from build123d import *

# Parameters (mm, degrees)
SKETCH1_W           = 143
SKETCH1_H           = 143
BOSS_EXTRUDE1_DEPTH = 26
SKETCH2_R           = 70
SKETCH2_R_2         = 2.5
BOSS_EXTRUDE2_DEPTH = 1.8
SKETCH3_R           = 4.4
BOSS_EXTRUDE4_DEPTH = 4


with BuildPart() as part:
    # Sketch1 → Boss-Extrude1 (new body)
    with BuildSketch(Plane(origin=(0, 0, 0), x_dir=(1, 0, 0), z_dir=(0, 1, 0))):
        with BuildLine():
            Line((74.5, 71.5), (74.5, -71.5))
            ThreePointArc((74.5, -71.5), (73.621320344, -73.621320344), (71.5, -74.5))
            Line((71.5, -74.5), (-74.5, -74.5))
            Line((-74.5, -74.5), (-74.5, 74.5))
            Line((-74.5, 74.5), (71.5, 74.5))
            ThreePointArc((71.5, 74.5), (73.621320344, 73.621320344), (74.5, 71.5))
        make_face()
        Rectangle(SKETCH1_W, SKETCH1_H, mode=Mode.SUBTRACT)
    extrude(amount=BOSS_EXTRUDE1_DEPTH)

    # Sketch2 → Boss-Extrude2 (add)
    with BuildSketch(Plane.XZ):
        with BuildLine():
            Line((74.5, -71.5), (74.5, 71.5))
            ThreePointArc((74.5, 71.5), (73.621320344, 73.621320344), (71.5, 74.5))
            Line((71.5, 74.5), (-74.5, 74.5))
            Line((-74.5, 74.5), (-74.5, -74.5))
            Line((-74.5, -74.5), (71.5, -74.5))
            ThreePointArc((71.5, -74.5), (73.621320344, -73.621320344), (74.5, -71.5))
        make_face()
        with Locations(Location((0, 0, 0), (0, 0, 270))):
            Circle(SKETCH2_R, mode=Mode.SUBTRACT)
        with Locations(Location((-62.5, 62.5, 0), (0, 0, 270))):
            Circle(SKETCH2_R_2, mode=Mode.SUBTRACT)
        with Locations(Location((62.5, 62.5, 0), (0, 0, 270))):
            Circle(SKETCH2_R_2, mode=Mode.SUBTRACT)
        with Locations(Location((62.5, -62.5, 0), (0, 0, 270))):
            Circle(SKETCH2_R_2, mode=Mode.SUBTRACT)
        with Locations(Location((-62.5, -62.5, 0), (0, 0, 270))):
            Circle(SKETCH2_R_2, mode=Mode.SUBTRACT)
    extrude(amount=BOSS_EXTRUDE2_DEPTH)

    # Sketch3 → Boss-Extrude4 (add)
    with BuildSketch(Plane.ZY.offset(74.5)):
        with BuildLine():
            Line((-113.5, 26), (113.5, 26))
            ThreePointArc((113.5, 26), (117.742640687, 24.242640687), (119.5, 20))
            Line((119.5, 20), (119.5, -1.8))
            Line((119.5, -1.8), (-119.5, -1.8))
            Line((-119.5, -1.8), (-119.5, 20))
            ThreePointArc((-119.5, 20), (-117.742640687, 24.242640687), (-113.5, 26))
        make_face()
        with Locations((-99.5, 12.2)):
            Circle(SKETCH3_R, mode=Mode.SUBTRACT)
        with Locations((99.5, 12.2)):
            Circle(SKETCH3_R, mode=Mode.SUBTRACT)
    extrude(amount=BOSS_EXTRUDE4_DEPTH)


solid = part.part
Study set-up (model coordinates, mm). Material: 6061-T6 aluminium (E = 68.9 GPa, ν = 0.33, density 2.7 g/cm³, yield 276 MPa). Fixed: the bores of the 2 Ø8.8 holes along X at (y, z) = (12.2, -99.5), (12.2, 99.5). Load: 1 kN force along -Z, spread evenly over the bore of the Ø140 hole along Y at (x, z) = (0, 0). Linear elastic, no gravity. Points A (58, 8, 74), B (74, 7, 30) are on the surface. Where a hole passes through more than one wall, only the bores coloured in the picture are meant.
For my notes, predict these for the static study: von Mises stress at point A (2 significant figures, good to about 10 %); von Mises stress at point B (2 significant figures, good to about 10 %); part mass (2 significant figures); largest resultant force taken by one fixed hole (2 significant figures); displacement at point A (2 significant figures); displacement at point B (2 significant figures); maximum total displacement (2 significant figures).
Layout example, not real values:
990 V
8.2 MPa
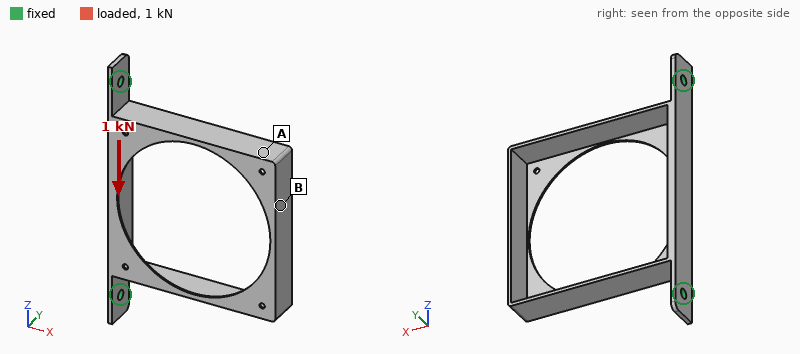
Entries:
16 MPa
34 MPa
230 g
670 N
1.4 mm
1.4 mm
1.6 mm
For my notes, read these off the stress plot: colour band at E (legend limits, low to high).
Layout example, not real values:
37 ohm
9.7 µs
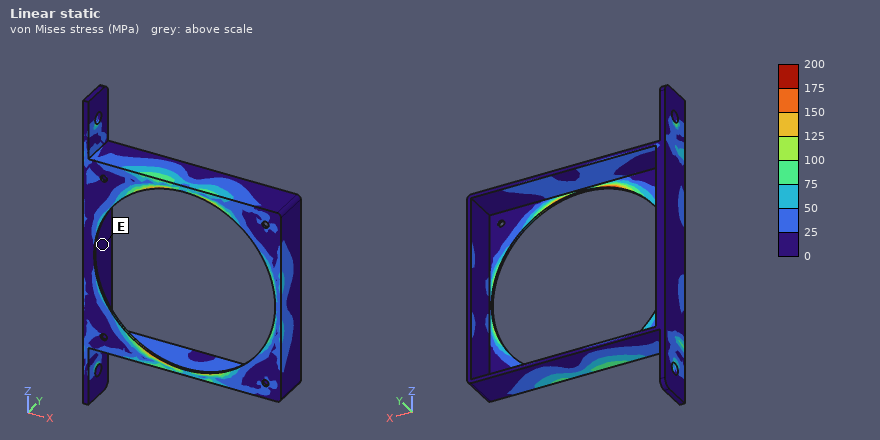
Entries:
0 to 25 MPa
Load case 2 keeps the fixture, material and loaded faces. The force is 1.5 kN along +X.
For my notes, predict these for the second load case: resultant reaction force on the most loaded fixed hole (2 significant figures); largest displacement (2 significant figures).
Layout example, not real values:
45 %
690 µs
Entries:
1.2 kN
2.0 mm
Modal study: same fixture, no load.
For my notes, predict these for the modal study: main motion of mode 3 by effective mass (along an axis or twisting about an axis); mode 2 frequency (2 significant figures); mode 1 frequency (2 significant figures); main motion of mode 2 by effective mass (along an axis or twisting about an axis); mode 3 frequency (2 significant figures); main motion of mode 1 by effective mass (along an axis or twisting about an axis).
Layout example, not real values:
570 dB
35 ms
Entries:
along Z
290 Hz
170 Hz
along Z
460 Hz
along Y
